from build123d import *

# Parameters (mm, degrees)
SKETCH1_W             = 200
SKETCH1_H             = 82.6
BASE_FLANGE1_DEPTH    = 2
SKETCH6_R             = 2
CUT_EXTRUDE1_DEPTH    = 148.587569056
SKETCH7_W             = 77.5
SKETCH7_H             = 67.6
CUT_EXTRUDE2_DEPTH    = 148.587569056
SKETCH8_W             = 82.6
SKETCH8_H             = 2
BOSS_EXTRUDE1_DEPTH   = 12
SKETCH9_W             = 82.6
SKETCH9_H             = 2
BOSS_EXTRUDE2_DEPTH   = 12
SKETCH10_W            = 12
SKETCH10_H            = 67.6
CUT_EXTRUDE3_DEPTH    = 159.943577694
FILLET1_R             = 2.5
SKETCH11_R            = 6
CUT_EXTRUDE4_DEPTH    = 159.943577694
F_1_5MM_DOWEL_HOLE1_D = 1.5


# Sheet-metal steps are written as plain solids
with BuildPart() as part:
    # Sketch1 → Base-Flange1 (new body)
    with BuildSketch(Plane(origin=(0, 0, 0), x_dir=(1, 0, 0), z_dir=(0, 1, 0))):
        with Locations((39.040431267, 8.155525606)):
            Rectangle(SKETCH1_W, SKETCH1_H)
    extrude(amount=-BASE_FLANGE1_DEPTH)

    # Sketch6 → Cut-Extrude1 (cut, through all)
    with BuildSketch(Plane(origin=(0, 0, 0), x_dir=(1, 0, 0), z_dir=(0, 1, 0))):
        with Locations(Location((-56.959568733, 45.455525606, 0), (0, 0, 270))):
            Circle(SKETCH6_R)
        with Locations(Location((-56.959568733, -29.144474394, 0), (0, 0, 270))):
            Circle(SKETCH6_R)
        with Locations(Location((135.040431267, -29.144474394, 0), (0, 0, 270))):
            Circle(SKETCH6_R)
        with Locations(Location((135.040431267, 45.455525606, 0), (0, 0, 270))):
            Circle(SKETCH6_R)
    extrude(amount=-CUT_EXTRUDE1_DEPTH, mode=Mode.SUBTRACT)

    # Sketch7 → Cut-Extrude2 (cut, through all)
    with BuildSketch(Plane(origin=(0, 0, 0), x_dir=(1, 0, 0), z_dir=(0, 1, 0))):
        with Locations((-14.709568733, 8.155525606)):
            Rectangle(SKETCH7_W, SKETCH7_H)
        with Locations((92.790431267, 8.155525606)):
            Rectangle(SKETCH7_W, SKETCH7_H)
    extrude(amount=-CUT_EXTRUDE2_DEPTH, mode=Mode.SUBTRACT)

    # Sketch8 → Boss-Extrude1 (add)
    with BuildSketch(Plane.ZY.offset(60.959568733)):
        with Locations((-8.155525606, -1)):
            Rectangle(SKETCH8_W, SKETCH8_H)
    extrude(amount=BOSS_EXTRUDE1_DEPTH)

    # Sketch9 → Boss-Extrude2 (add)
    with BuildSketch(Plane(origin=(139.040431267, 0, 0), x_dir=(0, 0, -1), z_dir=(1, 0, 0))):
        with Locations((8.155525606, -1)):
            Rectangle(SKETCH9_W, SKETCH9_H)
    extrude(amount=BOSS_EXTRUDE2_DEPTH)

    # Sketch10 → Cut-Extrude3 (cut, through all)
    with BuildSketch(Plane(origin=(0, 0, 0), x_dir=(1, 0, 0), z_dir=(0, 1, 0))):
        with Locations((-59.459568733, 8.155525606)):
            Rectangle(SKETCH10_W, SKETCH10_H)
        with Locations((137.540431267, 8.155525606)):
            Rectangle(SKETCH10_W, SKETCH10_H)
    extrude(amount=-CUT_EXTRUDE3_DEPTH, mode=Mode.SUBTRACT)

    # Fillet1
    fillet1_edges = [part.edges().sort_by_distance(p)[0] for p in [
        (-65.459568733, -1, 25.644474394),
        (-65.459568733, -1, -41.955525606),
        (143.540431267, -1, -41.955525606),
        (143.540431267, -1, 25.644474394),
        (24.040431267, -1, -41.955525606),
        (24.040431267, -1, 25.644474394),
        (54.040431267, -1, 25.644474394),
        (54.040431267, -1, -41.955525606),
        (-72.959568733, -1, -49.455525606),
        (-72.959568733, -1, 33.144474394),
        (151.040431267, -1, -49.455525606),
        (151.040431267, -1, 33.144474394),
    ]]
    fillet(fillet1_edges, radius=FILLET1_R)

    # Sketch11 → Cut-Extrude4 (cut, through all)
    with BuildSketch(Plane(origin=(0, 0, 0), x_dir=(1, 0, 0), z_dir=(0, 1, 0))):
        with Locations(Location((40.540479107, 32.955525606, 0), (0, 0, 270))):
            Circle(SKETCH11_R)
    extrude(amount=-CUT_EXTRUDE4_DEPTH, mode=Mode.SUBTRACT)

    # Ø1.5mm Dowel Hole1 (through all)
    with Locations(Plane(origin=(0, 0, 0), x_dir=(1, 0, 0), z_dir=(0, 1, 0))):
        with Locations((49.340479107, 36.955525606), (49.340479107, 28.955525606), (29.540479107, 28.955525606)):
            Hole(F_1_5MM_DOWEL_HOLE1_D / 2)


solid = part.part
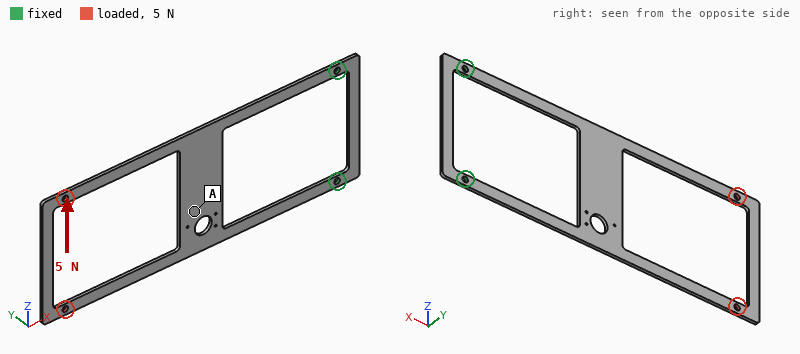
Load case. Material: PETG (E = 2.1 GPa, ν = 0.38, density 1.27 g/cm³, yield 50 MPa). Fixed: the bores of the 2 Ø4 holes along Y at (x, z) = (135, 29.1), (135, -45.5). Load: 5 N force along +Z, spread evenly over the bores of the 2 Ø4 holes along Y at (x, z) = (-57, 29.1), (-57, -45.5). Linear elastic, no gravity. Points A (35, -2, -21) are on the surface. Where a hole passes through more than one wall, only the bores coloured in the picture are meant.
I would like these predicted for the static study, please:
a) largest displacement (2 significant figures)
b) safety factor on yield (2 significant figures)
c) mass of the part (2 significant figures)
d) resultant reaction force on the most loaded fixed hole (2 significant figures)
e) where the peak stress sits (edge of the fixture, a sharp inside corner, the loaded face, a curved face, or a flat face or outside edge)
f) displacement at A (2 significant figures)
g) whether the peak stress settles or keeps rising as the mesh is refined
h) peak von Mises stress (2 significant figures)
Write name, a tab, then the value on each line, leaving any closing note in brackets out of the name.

largest displacement	2.5 mm
safety factor on yield	5.6
mass of the part	16 g
resultant reaction force on the most loaded fixed hole	10 N
where the peak stress sits	a curved face
displacement at A	0.91 mm
whether the peak stress settles or keeps rising as the mesh is refined	settles
peak von Mises stress	8.9 MPa
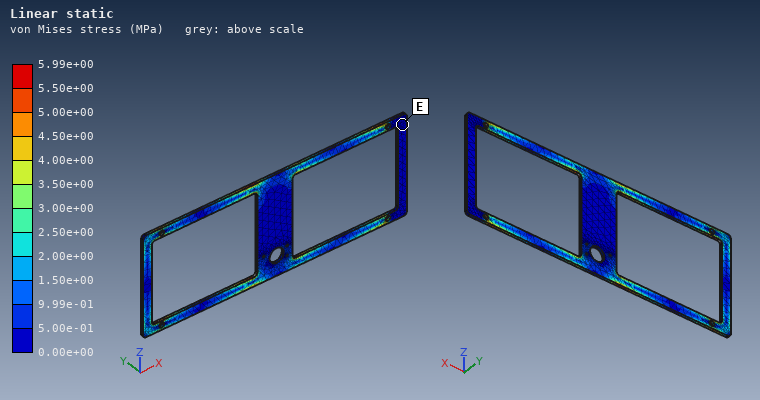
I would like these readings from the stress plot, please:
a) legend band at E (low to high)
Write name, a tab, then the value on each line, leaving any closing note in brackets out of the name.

legend band at E	0.00e+00 to 5.00e-01 MPa
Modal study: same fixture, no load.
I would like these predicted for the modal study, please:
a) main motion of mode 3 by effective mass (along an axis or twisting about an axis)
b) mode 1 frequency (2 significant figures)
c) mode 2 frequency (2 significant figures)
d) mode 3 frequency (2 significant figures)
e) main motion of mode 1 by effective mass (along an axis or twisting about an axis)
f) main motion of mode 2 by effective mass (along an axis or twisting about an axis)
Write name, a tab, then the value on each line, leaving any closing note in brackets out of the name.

main motion of mode 3 by effective mass	along Y
mode 1 frequency	7.4 Hz
mode 2 frequency	36 Hz
mode 3 frequency	40 Hz
main motion of mode 1 by effective mass	along Y
main motion of mode 2 by effective mass	twisting about X
